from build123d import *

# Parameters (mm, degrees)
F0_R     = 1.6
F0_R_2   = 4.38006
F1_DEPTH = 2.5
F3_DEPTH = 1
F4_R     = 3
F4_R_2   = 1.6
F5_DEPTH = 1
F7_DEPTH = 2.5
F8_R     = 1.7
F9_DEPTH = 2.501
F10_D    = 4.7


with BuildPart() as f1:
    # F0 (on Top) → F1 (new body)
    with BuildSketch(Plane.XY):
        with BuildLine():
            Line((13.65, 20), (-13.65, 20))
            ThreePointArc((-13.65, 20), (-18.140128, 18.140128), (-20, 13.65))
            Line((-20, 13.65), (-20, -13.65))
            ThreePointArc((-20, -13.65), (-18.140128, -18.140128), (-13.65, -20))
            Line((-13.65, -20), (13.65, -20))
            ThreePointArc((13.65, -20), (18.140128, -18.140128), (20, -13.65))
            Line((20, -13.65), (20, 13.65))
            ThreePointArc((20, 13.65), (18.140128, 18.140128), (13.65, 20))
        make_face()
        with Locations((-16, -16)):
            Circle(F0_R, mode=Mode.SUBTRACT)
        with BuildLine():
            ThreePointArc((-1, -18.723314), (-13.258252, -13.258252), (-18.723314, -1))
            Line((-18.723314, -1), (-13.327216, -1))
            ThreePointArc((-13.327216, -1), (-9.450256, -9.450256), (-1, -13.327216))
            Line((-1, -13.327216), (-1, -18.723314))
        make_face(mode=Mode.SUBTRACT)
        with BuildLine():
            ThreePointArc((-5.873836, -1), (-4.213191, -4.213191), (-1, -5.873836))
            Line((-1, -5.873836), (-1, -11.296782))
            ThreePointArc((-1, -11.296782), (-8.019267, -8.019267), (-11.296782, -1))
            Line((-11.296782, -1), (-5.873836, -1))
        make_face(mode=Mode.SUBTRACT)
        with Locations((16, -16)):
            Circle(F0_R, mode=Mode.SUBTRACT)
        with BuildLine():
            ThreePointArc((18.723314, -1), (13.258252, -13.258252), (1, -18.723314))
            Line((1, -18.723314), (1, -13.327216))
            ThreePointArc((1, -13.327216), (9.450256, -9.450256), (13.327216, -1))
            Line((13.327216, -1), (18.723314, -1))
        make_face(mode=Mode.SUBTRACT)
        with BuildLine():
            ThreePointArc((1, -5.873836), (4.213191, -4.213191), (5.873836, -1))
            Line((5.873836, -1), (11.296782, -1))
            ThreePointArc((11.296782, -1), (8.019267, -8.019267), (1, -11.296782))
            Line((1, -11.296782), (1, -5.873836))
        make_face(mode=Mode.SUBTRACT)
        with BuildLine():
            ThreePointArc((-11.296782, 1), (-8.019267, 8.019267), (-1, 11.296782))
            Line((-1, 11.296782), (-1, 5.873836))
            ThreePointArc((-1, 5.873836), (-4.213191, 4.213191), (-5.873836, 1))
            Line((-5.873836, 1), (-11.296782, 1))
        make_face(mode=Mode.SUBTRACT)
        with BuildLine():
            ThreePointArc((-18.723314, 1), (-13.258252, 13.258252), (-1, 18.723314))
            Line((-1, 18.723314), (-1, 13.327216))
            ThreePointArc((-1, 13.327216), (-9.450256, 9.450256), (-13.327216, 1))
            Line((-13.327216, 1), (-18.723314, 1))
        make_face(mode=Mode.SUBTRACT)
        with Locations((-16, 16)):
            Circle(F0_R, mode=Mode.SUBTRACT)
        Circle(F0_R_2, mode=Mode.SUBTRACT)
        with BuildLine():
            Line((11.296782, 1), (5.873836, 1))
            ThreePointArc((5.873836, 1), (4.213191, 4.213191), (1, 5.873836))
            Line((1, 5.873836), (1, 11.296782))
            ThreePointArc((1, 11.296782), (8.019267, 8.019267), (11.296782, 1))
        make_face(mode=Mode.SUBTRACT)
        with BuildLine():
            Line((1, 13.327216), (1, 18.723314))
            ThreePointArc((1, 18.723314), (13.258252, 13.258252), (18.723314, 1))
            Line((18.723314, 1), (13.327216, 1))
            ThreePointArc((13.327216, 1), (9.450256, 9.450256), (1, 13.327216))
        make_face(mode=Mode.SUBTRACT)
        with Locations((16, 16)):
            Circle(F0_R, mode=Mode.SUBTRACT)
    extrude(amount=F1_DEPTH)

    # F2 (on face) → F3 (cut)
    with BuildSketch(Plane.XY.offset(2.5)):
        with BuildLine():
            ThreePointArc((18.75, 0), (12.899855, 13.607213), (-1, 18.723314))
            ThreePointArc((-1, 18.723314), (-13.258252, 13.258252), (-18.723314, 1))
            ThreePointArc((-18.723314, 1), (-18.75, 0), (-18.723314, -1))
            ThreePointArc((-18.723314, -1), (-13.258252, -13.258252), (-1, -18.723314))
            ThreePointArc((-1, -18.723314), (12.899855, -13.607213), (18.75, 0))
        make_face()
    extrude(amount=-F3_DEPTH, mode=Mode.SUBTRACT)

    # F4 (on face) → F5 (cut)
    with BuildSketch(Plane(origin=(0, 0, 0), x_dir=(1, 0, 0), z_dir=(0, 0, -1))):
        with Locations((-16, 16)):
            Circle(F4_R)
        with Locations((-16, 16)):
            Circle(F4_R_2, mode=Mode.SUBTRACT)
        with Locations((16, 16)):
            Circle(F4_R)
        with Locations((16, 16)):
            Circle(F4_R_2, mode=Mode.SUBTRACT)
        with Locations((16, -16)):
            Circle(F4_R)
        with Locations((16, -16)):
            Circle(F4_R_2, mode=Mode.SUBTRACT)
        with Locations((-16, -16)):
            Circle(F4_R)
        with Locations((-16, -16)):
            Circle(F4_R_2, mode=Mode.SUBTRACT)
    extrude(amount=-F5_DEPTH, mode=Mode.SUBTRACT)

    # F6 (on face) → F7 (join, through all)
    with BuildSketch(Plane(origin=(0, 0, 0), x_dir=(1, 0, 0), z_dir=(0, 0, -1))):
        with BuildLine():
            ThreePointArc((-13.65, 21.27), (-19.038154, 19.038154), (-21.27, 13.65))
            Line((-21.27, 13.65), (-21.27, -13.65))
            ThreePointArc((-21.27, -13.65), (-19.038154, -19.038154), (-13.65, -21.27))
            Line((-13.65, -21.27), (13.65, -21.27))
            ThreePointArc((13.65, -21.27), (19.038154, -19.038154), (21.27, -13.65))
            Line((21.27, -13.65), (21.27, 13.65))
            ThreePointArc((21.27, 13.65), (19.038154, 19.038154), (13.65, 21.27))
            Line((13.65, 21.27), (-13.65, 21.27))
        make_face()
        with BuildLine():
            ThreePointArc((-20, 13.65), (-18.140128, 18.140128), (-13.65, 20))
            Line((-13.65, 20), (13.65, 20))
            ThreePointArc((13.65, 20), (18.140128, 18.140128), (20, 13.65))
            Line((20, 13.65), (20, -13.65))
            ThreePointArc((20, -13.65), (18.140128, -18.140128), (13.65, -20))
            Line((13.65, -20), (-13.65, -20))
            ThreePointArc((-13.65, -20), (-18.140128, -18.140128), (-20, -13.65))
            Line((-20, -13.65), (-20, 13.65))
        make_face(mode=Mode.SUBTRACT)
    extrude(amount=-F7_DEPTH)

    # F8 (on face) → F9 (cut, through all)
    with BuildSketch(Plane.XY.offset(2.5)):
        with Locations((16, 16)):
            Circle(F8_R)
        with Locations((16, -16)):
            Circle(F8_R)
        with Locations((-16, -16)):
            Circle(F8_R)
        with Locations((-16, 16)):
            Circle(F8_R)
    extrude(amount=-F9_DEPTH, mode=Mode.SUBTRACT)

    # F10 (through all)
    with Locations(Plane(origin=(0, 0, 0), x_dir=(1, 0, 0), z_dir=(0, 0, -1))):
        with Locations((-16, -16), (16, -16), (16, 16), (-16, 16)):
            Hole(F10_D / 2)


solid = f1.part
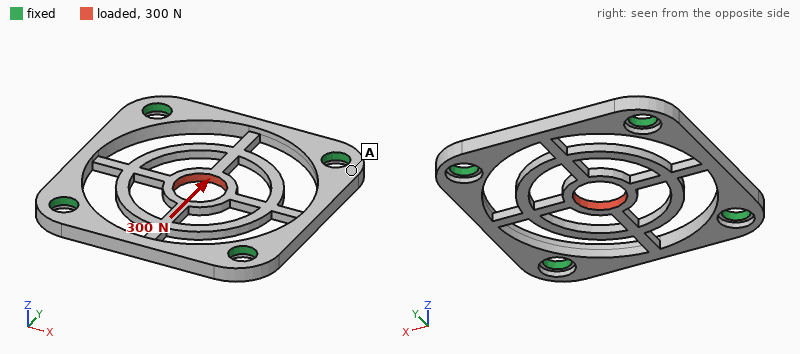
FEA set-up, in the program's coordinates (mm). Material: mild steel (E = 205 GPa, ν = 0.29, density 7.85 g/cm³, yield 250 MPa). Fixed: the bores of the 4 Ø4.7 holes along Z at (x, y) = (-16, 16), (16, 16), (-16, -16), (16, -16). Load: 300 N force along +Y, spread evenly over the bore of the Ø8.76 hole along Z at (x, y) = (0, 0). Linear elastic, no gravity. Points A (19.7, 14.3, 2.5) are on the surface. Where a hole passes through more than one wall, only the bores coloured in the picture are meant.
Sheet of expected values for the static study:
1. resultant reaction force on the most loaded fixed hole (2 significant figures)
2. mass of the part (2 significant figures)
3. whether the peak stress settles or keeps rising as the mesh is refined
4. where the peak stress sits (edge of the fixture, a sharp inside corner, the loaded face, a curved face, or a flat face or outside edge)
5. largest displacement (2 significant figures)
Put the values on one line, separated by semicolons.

110 N; 15 g; keeps rising; a sharp inside corner; 12 µm
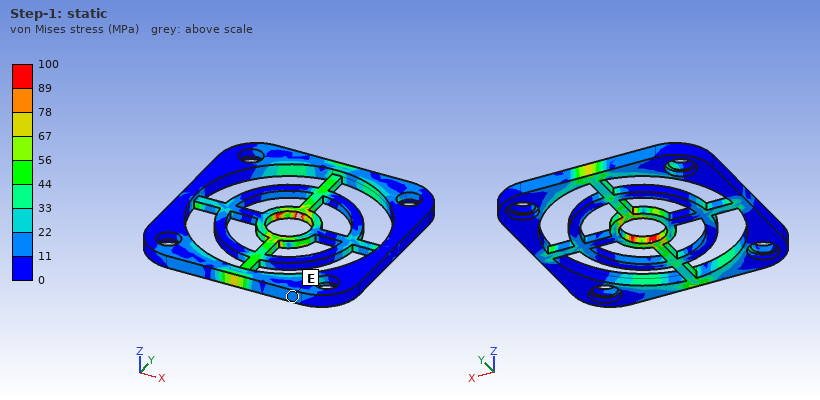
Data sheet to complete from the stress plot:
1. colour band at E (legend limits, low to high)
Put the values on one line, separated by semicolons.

11 to 22 MPa
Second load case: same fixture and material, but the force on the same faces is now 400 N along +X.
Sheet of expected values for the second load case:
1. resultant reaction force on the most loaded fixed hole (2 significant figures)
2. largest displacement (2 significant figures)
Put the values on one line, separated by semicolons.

140 N; 15 µm
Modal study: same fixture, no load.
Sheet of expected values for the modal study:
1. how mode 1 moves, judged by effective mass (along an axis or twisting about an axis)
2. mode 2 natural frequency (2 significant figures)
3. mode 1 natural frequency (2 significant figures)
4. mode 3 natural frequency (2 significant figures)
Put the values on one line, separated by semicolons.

along Z; 8000 Hz; 4800 Hz; 8000 Hz
